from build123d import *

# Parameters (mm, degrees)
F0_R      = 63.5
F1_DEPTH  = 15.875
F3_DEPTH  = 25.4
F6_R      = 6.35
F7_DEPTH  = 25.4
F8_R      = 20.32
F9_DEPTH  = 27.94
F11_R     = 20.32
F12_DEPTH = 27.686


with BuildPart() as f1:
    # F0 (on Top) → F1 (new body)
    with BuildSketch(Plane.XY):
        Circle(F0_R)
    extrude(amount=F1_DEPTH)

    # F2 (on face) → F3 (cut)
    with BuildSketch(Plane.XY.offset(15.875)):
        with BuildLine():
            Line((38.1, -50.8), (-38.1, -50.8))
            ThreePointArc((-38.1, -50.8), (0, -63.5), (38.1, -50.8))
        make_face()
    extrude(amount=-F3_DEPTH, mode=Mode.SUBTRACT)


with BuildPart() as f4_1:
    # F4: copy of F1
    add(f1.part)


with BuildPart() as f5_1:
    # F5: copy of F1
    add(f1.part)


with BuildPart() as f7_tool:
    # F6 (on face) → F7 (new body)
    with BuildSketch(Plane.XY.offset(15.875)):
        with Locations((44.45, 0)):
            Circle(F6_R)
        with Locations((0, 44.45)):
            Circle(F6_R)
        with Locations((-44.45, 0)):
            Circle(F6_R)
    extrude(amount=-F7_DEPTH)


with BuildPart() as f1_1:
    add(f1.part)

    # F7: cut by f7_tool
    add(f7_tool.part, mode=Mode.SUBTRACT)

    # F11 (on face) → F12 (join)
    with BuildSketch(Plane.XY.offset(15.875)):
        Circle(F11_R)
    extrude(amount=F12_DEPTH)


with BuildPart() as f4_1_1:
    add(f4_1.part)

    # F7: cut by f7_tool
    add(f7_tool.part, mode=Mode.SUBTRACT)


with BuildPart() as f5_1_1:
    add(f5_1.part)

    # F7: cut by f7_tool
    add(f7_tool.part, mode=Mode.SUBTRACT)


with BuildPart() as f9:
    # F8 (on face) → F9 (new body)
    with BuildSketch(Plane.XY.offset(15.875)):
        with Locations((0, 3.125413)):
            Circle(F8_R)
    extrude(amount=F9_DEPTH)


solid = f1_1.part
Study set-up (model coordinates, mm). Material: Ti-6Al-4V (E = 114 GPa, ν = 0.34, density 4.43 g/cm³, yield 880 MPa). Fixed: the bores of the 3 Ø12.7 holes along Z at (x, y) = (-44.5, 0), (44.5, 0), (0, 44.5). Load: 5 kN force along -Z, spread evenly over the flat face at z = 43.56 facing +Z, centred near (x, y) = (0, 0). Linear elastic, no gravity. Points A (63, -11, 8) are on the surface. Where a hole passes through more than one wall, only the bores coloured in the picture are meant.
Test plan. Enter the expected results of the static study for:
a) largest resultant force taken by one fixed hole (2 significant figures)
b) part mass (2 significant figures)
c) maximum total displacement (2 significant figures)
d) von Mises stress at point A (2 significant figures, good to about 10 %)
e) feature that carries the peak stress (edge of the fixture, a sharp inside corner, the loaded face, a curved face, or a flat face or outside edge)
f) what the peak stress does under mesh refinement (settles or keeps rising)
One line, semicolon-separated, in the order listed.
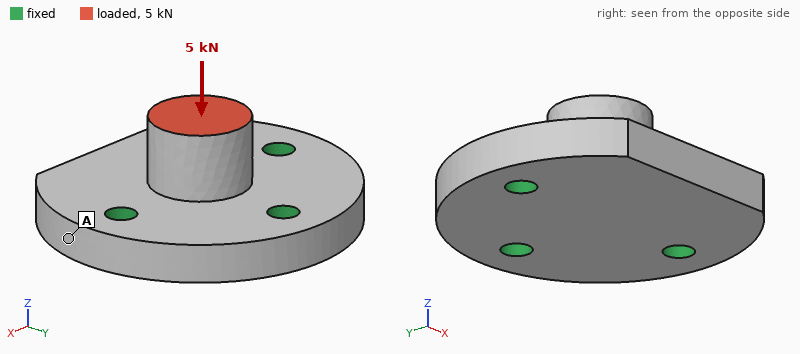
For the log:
2.0 kN; 980 g; 8.9 µm; 3.1 MPa; edge of the fixture; keeps rising
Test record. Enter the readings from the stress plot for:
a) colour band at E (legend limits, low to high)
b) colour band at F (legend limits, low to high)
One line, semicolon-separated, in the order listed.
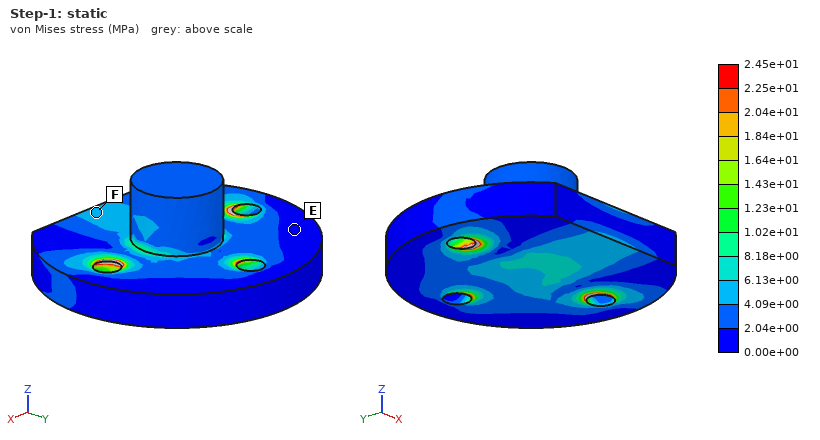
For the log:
0.00e+00 to 2.04e+00 MPa; 4.09e+00 to 6.13e+00 MPa
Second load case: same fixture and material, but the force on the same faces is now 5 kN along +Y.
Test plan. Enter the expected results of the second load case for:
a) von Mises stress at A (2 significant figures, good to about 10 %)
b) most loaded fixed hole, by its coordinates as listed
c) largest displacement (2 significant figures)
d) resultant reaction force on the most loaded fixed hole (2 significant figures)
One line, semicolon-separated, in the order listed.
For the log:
5.3 MPa; (0, 44.5); 24 µm; 3.8 kN
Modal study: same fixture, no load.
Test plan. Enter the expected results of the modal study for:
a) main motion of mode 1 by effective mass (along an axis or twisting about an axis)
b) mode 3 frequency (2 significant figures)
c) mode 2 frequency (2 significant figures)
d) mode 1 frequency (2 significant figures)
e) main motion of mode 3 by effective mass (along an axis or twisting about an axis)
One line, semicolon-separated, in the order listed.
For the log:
along Z; 10 kHz; 8500 Hz; 4500 Hz; along Z
